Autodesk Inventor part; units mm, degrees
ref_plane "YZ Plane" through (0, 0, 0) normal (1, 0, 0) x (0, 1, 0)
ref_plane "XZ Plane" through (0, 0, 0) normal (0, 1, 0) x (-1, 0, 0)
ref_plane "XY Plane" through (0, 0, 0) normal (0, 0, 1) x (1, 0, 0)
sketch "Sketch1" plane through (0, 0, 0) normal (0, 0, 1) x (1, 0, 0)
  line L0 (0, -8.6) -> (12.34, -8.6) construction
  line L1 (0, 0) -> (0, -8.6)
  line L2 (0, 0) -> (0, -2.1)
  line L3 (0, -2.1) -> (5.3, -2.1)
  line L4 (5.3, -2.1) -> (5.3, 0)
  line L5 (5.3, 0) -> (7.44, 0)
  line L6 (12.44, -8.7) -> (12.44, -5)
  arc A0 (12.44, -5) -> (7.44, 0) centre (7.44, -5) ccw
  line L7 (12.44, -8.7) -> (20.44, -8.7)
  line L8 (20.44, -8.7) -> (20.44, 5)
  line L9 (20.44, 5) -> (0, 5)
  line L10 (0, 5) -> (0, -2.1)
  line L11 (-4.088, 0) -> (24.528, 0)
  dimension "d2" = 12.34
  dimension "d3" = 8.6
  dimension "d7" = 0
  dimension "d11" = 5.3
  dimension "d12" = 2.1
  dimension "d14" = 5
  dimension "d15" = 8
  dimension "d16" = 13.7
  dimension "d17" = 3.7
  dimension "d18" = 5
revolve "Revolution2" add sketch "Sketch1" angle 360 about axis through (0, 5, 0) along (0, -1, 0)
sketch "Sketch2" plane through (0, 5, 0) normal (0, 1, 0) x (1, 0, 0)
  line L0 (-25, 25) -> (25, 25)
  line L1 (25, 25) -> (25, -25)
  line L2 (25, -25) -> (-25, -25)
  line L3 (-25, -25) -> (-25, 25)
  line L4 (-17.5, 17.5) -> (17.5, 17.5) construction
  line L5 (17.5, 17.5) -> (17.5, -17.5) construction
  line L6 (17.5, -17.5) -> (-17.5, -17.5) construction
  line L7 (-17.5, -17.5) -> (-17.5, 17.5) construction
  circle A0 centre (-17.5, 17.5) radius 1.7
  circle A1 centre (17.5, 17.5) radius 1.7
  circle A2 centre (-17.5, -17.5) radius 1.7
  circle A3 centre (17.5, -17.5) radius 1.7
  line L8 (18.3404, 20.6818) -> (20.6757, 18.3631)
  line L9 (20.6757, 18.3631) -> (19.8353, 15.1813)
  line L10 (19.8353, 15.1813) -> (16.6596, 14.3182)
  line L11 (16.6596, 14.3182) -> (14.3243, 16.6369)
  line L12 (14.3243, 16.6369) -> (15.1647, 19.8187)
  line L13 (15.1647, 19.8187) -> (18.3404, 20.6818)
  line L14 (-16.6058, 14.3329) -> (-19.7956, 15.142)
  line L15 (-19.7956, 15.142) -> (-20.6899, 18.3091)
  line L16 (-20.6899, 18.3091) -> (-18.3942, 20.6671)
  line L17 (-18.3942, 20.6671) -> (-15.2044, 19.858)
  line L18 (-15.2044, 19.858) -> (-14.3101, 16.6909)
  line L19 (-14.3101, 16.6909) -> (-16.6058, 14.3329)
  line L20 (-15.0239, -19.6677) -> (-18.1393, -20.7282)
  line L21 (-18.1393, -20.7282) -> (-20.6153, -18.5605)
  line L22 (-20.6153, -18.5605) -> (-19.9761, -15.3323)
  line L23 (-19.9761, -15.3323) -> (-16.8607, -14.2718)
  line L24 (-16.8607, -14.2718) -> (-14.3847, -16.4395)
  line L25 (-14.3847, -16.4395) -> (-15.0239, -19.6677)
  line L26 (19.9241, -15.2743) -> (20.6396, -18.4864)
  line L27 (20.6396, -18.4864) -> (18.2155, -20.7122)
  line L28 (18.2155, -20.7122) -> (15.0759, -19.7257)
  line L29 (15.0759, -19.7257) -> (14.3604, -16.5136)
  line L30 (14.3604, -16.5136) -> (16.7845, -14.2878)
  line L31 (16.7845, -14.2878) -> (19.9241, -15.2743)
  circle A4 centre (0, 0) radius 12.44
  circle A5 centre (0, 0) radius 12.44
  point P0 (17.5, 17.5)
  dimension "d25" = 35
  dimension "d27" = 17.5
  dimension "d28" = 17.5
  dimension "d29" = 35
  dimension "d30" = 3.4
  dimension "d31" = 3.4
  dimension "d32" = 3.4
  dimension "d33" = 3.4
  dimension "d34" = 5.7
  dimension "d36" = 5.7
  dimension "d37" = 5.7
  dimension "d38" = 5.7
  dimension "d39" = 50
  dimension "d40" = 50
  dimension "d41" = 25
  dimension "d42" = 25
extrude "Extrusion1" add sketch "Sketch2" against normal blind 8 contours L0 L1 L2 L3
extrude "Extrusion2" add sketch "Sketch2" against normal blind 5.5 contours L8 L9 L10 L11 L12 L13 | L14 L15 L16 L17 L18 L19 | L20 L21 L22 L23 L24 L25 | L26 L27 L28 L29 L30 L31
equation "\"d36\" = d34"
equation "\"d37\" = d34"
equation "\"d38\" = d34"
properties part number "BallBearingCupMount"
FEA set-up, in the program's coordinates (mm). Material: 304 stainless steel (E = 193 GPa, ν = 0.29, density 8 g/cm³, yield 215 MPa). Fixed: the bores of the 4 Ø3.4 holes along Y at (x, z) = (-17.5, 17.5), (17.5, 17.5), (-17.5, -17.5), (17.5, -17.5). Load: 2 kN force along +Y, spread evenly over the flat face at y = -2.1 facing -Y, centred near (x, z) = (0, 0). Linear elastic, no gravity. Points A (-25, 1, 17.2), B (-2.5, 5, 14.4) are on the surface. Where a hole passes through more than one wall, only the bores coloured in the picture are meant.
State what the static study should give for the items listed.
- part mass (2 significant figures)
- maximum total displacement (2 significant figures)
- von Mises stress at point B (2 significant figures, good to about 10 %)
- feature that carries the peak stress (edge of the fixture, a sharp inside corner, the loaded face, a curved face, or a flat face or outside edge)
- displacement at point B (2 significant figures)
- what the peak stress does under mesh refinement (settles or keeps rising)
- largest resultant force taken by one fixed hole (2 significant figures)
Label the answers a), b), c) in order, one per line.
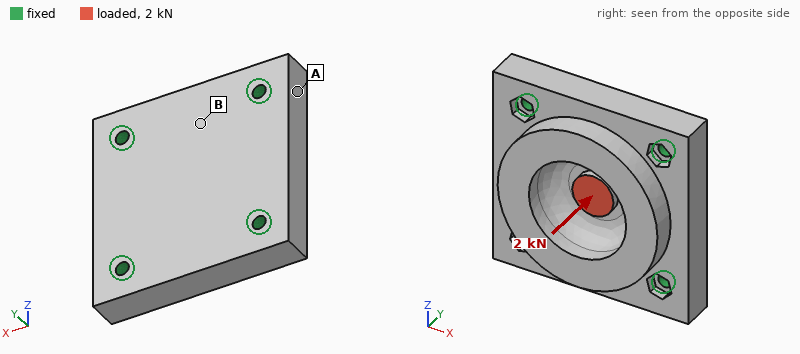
a) 190 g
b) 5.1 µm
c) 9.9 MPa
d) edge of the fixture
e) 1.8 µm
f) keeps rising
g) 570 N
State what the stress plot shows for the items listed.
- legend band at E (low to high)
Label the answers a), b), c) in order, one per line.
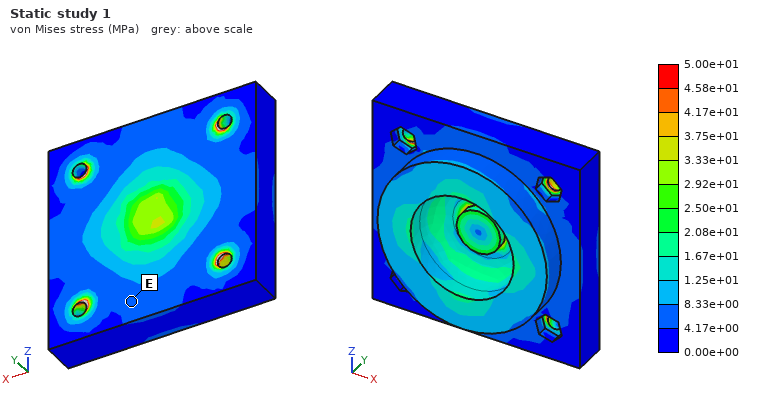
a) 4.17e+00 to 8.33e+00 MPa
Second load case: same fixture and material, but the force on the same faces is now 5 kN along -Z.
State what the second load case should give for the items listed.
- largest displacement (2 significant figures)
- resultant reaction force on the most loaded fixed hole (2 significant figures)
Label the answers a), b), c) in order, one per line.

a) 9.8 µm
b) 1.4 kN
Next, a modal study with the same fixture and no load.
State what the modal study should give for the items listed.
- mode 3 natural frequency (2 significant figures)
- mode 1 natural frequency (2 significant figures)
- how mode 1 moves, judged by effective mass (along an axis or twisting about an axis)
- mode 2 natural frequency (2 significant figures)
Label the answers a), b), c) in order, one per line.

a) 23 kHz
b) 18 kHz
c) along Y
d) 22 kHz
